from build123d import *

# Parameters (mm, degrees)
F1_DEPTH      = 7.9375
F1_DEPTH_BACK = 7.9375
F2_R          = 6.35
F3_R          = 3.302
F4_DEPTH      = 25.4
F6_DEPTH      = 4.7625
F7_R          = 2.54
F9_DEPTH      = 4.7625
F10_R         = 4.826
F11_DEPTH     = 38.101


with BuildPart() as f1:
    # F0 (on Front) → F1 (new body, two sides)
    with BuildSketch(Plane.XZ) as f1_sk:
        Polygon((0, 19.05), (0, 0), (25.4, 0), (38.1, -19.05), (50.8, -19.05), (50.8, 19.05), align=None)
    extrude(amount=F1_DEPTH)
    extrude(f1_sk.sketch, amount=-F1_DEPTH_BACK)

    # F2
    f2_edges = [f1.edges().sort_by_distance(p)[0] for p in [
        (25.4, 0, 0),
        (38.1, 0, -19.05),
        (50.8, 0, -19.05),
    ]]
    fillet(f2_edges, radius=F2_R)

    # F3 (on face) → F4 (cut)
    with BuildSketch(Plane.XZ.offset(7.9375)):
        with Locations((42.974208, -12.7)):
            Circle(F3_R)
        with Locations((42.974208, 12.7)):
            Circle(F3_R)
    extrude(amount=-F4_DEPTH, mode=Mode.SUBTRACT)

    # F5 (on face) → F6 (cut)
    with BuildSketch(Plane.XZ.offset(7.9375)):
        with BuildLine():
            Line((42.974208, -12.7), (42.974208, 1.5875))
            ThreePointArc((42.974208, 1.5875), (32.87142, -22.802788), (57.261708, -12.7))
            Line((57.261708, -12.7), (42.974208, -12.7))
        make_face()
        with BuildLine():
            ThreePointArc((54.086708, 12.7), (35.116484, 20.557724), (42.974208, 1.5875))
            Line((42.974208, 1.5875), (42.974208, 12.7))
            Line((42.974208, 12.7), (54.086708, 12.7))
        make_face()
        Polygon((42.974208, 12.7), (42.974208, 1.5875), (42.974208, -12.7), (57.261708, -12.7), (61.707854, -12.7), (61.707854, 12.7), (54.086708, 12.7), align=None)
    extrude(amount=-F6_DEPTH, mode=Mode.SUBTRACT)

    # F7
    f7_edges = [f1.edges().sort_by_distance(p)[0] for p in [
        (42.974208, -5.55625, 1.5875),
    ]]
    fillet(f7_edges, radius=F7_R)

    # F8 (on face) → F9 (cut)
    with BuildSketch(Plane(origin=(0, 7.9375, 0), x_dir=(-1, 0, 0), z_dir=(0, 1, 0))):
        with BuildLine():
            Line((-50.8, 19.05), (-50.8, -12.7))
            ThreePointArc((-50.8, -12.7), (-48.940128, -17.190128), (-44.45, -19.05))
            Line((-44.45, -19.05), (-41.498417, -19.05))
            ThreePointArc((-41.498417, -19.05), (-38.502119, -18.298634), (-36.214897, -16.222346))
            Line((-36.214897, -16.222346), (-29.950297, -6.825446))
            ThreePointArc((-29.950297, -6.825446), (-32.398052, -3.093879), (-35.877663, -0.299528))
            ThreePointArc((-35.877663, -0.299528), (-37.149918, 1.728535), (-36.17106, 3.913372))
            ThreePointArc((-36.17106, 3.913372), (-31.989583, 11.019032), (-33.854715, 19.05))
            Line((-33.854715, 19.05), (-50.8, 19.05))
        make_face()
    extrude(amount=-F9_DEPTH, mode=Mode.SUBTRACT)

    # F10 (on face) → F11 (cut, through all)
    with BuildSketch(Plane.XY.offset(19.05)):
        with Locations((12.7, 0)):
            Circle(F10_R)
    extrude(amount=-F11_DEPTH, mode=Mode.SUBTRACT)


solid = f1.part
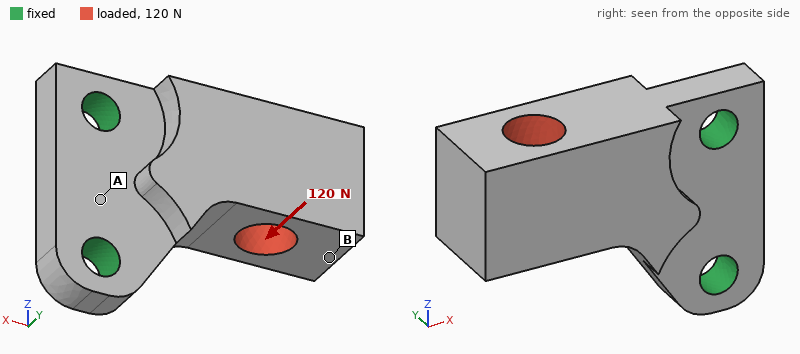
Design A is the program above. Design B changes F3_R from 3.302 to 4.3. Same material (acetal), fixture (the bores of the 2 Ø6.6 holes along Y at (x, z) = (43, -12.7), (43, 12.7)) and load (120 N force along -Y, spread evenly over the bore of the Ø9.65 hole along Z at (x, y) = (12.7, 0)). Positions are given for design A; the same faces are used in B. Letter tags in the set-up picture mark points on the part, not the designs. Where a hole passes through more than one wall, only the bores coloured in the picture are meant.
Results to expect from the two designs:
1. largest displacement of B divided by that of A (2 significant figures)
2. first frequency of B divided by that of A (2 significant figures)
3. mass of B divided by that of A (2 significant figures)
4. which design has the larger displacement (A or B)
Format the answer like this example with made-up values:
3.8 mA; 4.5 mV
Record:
0.86; 1.1; 0.98; A
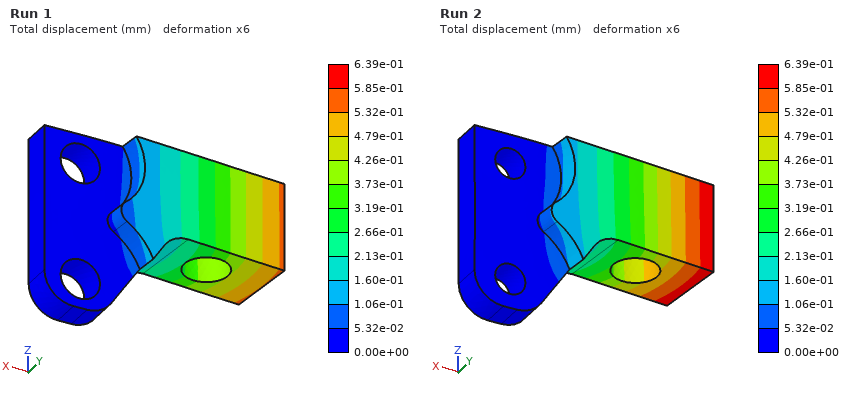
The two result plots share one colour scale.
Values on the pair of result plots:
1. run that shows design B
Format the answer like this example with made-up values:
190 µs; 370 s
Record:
Run 1
